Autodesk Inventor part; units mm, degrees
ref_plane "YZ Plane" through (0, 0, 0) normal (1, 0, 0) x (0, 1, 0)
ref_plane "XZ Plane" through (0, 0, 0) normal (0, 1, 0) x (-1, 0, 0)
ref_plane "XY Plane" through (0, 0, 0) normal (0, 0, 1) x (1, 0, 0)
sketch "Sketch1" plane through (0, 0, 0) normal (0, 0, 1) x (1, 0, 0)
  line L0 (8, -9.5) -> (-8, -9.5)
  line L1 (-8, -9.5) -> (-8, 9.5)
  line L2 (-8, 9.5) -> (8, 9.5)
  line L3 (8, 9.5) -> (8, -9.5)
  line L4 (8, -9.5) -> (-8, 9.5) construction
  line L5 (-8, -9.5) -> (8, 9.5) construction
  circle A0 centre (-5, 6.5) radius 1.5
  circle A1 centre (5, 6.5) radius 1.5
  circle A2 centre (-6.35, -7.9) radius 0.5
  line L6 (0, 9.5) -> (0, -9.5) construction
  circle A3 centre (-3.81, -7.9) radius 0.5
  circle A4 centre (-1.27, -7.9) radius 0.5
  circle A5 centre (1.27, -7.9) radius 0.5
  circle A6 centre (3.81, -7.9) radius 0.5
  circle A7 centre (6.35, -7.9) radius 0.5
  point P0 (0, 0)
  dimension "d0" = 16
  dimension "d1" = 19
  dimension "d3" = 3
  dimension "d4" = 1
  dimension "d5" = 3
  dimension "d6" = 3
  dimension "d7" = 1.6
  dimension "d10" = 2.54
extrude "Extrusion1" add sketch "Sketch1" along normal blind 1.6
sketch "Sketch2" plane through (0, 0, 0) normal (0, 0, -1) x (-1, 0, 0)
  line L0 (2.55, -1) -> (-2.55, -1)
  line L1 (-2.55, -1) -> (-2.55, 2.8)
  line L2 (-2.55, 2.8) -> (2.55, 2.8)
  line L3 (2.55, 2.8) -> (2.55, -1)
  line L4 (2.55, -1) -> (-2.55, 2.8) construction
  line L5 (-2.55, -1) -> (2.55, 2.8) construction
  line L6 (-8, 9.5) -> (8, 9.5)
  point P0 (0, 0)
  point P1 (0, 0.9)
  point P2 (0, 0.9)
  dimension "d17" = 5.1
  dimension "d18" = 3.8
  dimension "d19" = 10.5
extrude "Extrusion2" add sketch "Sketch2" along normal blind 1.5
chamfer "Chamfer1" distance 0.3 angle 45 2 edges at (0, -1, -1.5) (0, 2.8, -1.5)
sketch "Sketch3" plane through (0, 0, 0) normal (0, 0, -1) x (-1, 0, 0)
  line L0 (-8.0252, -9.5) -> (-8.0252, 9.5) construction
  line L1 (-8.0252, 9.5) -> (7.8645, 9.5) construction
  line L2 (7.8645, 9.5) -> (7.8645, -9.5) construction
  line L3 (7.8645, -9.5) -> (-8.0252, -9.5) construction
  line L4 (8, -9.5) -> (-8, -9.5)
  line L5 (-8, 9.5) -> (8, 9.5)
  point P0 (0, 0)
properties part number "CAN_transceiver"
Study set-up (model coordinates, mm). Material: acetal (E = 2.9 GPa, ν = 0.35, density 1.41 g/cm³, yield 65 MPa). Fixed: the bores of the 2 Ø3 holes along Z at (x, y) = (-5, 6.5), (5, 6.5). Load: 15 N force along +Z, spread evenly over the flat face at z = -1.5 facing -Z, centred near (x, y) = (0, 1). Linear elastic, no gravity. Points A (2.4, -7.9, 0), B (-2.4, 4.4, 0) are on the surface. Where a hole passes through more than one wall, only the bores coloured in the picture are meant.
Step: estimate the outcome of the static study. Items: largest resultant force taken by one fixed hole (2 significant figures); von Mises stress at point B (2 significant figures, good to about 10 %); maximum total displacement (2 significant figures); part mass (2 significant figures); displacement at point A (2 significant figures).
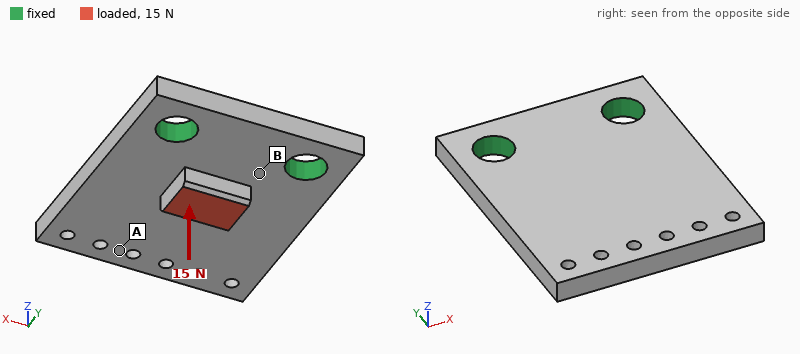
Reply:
7.5 N
5.5 MPa
0.16 mm
0.68 g
0.14 mm
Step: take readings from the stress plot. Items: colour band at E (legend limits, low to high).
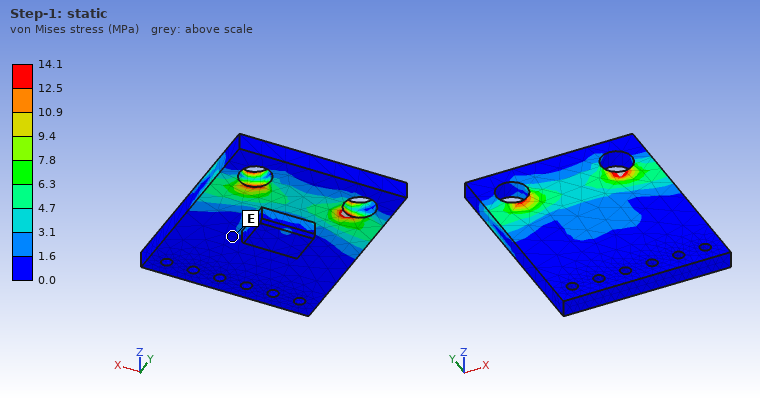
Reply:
0.0 to 1.6 MPa
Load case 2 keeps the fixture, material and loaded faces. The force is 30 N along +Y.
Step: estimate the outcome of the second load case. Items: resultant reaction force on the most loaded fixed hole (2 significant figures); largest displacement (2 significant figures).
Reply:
16 N
0.23 mm
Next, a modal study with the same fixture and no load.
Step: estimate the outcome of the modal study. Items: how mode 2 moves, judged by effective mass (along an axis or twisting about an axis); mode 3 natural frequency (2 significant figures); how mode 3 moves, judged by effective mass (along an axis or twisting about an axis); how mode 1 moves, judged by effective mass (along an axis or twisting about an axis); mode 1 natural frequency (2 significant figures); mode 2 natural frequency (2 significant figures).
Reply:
twisting about Y
9500 Hz
along Z
along Z
1800 Hz
4100 Hz
